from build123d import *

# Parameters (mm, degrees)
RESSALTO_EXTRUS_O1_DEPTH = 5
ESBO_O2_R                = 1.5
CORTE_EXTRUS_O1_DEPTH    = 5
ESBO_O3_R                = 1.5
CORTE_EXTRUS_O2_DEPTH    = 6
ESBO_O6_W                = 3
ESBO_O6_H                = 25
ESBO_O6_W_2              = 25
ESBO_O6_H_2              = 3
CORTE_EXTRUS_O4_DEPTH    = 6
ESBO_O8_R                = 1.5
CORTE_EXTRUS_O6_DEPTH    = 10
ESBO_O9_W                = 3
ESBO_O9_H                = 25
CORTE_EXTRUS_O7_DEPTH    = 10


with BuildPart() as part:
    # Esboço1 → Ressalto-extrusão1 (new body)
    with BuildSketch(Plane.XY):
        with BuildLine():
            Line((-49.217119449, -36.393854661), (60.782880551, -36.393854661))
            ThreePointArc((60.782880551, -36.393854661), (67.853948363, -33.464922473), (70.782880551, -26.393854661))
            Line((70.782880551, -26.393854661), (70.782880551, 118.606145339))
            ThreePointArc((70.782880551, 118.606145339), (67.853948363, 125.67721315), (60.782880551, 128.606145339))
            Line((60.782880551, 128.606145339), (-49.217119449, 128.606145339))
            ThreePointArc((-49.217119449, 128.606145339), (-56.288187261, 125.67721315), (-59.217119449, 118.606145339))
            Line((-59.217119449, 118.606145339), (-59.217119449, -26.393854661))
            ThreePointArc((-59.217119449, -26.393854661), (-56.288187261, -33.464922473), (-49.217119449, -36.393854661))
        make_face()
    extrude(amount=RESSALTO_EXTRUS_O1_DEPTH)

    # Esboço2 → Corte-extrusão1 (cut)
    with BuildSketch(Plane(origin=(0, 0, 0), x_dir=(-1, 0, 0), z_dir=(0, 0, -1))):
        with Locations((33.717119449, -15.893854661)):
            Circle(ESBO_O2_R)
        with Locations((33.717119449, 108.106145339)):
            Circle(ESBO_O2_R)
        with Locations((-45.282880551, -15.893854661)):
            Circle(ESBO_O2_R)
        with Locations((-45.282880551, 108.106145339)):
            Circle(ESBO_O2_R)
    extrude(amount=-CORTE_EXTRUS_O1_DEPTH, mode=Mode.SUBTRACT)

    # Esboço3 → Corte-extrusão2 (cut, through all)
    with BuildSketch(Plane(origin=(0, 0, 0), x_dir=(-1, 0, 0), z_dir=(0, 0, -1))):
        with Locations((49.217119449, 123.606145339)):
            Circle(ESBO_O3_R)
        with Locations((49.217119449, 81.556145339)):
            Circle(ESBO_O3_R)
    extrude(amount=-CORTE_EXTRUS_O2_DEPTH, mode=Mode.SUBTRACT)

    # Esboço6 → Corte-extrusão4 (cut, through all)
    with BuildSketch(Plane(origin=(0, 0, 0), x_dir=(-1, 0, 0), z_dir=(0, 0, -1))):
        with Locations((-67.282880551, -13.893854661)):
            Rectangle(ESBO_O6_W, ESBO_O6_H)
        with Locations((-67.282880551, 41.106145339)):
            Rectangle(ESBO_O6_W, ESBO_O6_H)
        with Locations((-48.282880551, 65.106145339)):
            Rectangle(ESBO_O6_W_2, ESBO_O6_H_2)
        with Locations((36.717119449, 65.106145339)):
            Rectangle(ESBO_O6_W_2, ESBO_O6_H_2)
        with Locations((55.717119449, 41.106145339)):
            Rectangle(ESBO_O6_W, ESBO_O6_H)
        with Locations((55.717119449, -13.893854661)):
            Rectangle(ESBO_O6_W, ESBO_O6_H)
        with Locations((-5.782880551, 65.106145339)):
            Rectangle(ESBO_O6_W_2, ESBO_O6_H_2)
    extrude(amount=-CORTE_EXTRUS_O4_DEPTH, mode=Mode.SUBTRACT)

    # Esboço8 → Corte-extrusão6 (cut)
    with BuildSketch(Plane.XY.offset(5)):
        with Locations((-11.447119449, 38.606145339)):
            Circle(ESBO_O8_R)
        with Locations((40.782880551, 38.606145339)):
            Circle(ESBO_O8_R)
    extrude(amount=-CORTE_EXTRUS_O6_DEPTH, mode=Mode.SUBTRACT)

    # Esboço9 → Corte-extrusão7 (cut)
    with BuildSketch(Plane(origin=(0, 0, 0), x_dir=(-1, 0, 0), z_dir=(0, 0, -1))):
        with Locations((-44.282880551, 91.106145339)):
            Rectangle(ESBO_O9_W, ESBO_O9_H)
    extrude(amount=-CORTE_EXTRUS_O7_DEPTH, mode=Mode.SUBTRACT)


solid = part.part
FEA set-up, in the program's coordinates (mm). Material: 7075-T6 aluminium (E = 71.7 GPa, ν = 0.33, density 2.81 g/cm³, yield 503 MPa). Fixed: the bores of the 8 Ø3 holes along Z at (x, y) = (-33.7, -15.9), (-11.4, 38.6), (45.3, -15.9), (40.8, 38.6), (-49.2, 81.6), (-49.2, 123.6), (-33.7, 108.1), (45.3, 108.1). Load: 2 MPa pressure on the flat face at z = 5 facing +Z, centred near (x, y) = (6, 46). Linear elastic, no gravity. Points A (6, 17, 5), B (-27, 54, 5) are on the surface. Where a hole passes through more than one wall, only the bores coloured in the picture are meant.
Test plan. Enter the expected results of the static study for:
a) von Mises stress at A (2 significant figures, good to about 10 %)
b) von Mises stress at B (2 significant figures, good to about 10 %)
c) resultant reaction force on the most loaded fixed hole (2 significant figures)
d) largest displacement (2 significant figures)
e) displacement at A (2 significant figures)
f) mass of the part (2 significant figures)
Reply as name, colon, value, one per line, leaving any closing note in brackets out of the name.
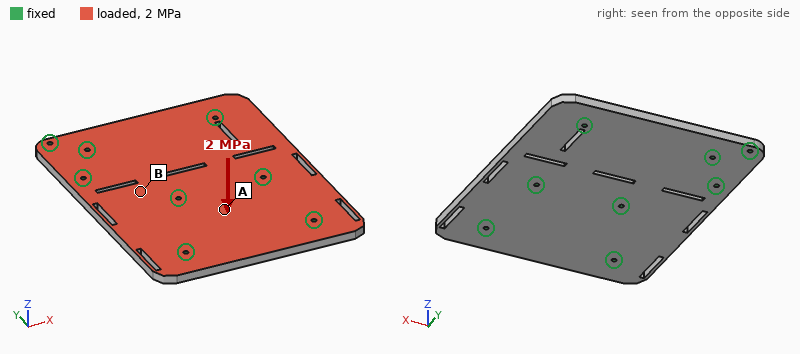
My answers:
von Mises stress at A: 41 MPa
von Mises stress at B: 140 MPa
resultant reaction force on the most loaded fixed hole: 7.5 kN
largest displacement: 0.53 mm
displacement at A: 0.15 mm
mass of the part: 290 g
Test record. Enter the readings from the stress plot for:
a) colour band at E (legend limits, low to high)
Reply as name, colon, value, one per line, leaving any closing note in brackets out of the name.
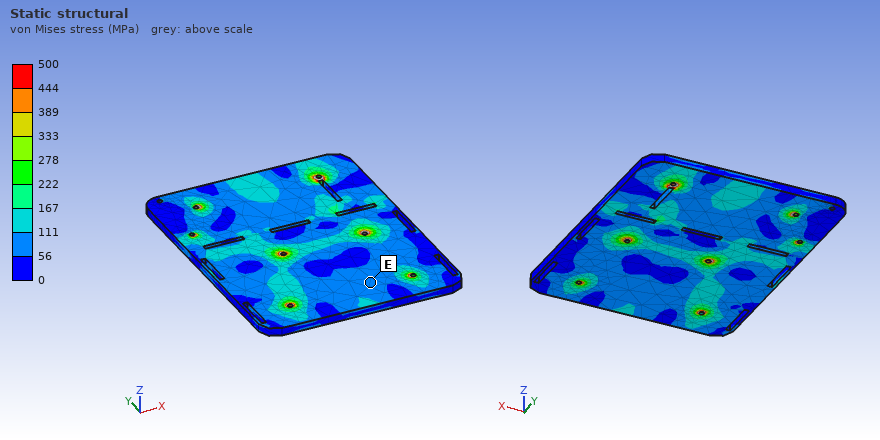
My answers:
colour band at E: 56 to 111 MPa
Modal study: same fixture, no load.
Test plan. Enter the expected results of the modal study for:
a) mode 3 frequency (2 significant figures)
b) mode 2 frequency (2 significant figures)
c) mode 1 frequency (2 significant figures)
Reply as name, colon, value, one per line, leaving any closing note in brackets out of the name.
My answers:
mode 3 frequency: 3300 Hz
mode 2 frequency: 3200 Hz
mode 1 frequency: 2900 Hz
